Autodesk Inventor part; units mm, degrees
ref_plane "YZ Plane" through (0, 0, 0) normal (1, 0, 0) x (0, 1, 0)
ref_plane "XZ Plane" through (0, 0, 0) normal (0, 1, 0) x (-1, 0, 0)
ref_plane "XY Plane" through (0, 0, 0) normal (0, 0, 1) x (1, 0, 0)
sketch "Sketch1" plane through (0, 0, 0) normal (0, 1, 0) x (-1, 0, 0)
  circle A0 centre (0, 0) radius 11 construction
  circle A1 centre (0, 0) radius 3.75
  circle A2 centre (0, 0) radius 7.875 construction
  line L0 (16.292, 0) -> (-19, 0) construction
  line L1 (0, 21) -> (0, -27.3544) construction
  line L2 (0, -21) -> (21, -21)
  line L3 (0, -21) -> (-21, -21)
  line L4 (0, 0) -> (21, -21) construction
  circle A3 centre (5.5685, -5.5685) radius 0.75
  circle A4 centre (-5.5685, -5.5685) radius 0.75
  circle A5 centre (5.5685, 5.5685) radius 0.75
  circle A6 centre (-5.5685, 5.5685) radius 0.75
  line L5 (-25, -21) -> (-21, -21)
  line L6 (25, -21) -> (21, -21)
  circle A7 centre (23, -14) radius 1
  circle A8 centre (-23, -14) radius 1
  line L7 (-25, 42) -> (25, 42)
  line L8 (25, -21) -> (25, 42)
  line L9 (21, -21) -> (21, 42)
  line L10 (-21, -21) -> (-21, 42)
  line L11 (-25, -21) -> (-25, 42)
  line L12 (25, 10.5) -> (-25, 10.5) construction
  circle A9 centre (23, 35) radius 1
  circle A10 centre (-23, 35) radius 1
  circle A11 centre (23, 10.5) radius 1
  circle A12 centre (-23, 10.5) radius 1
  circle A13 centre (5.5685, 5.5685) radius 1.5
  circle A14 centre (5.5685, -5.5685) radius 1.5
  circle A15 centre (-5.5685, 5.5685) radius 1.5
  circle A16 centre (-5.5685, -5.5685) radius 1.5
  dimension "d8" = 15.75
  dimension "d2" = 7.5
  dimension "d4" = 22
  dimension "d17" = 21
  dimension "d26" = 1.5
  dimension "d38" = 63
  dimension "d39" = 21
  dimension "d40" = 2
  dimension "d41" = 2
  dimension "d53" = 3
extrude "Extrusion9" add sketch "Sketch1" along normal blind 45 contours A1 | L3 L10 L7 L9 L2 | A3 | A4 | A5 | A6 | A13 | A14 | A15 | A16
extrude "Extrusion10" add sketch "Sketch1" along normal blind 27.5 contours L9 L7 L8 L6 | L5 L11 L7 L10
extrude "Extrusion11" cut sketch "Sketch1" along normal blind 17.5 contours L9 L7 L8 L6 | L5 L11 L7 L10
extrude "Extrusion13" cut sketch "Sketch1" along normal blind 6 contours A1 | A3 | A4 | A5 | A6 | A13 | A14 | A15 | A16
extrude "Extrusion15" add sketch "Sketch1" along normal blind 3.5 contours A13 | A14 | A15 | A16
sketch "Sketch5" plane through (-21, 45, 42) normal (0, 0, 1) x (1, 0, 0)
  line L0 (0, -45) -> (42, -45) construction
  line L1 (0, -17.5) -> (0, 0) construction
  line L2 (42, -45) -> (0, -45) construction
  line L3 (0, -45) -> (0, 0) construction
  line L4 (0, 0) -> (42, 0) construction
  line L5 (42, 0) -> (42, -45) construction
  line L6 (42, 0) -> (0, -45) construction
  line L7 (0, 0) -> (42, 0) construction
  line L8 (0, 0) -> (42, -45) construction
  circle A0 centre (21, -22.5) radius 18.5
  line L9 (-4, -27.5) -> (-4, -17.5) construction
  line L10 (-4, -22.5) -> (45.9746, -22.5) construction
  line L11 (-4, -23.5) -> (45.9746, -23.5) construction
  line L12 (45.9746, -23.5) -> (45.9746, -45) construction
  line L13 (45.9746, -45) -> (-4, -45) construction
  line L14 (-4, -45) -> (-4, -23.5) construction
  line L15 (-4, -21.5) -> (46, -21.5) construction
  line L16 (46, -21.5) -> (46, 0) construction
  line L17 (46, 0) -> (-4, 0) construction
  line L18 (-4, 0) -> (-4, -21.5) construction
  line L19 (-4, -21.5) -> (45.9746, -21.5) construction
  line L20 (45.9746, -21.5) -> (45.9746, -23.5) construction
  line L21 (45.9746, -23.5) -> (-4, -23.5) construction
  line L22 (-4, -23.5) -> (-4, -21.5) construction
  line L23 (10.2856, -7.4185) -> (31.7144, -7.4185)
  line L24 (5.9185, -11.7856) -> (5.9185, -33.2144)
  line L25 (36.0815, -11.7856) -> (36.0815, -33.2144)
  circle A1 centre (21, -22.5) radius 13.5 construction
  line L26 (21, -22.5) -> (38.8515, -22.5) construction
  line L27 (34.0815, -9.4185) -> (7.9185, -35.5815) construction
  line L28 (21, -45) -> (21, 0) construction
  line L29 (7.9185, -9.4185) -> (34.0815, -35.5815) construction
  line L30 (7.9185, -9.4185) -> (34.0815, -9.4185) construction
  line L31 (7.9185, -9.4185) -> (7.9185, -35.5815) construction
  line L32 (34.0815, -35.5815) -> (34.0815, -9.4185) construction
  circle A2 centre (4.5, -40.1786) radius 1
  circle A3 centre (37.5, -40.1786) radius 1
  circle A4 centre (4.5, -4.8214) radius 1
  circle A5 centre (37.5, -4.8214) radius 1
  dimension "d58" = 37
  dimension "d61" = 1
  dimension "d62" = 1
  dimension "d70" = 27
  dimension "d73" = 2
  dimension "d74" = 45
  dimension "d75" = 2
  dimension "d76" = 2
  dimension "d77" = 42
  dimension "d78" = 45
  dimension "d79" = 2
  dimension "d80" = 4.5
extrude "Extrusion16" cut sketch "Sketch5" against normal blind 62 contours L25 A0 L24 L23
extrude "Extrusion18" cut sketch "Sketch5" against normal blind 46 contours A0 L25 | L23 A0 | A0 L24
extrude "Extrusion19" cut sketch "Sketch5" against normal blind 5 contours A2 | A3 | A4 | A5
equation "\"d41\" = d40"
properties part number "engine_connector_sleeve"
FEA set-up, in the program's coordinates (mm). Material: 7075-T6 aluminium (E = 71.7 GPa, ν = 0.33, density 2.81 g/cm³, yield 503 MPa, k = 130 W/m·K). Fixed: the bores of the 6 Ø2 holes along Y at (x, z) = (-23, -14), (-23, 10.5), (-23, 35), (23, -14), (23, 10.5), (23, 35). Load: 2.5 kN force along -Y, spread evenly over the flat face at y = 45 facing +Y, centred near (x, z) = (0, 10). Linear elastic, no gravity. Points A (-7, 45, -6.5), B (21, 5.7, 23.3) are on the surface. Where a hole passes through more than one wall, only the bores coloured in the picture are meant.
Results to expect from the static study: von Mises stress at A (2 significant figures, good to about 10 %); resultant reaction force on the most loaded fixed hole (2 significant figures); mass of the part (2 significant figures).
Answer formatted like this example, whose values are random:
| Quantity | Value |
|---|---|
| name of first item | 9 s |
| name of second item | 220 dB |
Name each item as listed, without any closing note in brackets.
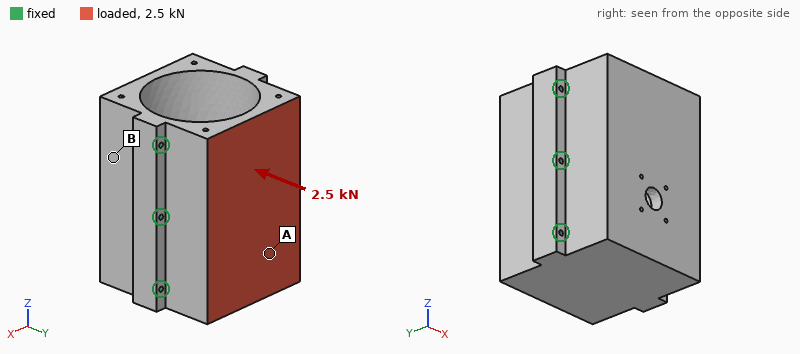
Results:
| Quantity | Value |
|---|---|
| von Mises stress at A | 3.2 MPa |
| resultant reaction force on the most loaded fixed hole | 490 N |
| mass of the part | 170 g |
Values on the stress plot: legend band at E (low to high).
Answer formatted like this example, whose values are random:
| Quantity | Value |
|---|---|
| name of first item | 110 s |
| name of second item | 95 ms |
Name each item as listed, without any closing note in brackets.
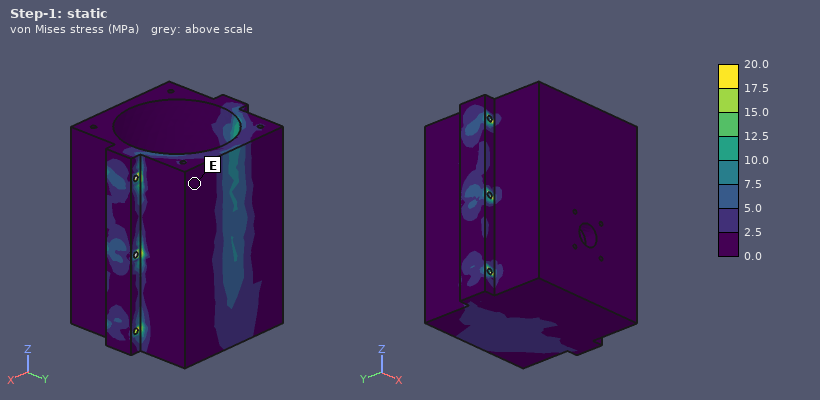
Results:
| Quantity | Value |
|---|---|
| legend band at E | 0.0 to 2.5 MPa |
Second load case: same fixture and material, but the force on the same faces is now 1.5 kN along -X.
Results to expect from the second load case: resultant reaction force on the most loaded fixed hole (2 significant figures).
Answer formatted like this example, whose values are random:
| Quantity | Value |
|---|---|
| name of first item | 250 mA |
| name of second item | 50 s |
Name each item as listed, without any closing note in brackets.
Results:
| Quantity | Value |
|---|---|
| resultant reaction force on the most loaded fixed hole | 440 N |
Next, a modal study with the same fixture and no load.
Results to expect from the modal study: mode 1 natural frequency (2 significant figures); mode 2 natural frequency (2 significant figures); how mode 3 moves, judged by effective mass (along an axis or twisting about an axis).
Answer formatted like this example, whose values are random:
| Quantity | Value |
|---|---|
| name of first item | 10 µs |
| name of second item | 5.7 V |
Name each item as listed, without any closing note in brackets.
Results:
| Quantity | Value |
|---|---|
| mode 1 natural frequency | 10 kHz |
| mode 2 natural frequency | 10 kHz |
| how mode 3 moves, judged by effective mass | along X |
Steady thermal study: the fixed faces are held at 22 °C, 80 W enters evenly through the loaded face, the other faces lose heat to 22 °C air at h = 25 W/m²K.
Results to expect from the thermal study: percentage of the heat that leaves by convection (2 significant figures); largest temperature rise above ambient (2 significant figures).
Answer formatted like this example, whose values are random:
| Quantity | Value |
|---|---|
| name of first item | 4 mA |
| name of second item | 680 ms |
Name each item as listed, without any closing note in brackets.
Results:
| Quantity | Value |
|---|---|
| percentage of the heat that leaves by convection | 4.5 % |
| largest temperature rise above ambient | 22 K |
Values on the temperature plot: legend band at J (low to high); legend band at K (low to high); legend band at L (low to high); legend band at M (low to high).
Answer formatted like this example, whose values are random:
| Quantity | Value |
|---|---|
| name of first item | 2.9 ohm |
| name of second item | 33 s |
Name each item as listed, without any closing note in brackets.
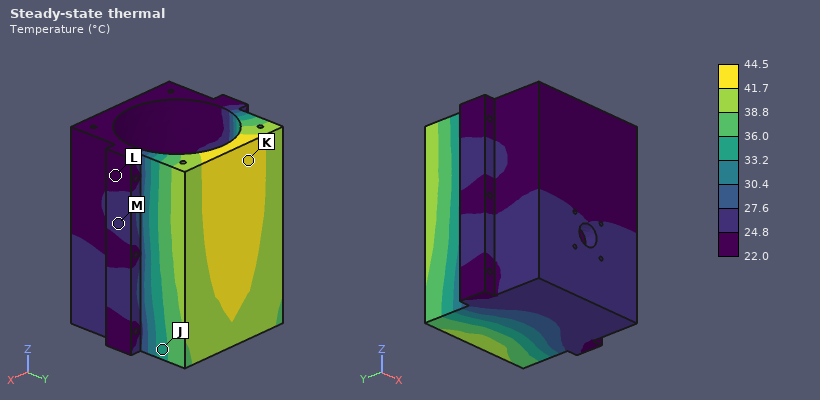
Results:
| Quantity | Value |
|---|---|
| legend band at J | 33.2 to 36.0 °C |
| legend band at K | 41.7 to 44.5 °C |
| legend band at L | 22.0 to 24.8 °C |
| legend band at M | 24.8 to 27.6 °C |
